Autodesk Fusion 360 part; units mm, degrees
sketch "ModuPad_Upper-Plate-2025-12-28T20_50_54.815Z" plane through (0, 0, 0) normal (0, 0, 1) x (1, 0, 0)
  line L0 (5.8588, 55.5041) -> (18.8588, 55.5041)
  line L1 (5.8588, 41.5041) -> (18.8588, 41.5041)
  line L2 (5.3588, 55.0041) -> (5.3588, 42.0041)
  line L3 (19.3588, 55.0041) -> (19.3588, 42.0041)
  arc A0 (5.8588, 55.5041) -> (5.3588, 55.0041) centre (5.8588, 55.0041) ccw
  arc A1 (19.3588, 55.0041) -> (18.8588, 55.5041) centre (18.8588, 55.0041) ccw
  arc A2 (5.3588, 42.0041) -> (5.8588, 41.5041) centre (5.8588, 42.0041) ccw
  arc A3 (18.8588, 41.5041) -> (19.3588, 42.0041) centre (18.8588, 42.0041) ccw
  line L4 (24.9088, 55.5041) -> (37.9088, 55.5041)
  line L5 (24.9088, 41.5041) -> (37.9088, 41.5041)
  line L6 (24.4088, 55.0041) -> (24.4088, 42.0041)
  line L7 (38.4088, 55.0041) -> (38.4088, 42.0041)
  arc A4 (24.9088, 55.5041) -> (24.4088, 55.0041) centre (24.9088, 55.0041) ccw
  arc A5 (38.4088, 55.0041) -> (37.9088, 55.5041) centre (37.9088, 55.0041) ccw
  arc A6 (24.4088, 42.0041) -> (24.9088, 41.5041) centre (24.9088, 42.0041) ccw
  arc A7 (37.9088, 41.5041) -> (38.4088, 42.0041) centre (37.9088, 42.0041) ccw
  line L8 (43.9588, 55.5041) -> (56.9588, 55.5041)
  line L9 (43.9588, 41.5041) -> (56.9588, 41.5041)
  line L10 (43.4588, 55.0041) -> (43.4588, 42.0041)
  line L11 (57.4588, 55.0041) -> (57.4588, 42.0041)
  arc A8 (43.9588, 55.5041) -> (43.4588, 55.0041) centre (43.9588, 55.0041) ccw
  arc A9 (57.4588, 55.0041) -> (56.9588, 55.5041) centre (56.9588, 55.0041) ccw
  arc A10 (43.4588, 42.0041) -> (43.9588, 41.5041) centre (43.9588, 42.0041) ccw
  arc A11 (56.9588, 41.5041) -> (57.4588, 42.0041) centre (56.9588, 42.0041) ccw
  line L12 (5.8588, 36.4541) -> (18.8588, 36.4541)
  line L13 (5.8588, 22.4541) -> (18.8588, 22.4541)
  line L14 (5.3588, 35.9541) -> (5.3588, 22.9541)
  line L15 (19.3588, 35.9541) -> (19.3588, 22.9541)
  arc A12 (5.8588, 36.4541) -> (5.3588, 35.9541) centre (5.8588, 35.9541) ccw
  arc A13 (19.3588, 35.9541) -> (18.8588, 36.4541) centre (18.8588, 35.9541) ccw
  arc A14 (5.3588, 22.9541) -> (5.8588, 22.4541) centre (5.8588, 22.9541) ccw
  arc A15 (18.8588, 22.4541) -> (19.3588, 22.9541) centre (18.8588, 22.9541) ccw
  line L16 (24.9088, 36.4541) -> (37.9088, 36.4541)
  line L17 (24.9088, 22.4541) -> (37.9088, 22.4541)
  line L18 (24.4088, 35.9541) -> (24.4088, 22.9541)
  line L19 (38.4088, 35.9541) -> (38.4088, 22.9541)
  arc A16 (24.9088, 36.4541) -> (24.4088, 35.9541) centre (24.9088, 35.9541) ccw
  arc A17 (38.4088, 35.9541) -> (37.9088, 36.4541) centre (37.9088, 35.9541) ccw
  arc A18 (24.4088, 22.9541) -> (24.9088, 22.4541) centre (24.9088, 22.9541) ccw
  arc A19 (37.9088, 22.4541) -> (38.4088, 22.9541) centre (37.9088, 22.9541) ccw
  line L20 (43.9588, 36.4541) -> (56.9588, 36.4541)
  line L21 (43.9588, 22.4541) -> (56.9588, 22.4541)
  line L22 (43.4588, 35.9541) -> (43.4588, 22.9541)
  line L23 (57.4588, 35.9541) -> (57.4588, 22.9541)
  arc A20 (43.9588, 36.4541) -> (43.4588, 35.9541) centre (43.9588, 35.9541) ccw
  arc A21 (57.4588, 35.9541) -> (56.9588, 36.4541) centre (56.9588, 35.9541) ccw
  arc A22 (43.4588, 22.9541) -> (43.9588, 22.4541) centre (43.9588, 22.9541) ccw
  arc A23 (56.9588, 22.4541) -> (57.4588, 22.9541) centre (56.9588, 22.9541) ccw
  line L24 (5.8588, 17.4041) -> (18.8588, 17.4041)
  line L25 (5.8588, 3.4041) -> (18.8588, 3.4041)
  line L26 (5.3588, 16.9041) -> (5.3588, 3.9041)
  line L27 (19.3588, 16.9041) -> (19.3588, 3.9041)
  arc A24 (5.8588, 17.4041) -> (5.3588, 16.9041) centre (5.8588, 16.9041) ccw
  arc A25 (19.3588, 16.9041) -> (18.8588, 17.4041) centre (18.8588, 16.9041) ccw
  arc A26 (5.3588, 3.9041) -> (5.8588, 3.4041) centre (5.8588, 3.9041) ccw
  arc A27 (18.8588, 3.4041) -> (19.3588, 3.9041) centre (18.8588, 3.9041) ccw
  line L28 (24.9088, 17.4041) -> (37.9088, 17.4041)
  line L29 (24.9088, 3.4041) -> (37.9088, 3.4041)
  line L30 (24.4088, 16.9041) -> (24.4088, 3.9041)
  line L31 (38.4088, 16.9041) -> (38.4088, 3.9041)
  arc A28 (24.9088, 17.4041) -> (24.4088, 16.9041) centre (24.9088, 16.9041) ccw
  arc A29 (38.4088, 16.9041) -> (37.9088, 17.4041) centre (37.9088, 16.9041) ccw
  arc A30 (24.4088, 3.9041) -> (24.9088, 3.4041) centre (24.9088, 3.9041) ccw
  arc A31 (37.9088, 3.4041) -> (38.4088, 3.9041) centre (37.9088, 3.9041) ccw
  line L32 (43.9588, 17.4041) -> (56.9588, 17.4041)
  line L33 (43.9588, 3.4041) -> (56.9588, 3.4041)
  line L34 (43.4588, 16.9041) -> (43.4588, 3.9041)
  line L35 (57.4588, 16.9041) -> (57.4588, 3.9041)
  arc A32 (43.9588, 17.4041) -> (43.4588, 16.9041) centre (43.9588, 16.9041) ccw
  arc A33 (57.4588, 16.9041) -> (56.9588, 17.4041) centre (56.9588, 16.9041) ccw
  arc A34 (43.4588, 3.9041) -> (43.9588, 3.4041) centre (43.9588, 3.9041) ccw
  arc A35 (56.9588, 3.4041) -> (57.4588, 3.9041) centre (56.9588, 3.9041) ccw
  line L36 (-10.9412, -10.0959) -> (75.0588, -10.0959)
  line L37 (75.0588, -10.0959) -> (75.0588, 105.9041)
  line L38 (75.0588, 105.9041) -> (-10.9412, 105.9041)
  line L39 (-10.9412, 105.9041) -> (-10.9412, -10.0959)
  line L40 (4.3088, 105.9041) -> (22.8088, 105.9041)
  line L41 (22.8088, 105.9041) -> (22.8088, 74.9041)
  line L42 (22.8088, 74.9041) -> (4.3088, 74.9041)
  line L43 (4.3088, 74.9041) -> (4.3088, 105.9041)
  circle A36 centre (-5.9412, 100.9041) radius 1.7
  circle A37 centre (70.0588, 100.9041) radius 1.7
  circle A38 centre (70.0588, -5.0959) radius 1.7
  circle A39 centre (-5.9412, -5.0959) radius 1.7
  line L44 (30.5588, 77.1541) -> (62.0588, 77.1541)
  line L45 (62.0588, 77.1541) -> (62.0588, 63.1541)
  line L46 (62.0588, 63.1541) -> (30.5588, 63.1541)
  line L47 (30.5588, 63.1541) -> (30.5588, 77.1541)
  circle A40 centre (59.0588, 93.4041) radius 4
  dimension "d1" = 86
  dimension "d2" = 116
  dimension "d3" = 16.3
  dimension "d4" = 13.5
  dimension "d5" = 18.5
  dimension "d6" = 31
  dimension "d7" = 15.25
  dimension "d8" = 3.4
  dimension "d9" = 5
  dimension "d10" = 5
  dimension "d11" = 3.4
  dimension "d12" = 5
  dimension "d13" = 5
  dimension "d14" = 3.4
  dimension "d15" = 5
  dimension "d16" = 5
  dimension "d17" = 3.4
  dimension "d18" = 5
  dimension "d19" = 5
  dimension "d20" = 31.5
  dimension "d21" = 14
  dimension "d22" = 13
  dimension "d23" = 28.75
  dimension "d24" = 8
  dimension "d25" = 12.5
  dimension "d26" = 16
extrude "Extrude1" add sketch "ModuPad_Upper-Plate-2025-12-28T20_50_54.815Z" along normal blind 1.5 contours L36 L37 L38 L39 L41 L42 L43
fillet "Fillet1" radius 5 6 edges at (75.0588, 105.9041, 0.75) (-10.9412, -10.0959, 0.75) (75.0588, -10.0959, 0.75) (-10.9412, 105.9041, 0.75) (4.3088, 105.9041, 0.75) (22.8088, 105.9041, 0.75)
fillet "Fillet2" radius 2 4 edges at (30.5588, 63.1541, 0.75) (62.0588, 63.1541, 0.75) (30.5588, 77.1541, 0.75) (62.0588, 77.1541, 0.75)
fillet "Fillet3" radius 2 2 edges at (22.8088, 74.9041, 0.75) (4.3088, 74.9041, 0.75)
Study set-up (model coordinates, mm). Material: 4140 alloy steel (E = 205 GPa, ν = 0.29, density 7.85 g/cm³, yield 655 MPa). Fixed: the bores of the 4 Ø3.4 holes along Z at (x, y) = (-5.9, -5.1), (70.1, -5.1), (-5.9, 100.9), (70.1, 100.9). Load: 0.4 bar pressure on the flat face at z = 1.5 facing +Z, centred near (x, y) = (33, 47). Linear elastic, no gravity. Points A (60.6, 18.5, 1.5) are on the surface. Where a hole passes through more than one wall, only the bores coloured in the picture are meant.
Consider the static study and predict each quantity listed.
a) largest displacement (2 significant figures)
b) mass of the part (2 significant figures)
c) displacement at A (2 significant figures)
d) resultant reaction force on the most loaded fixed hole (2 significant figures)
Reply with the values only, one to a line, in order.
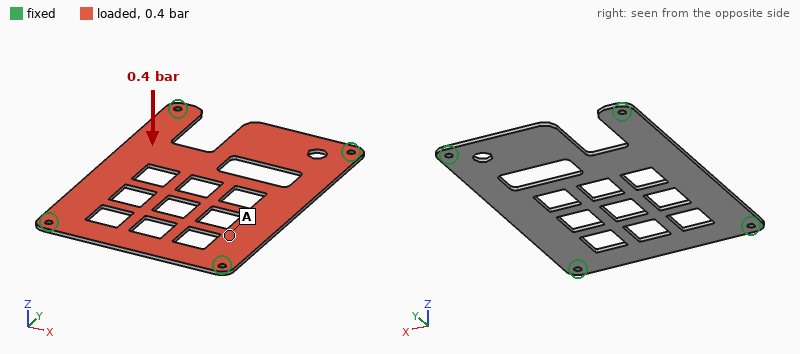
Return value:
0.44 mm
83 g
0.18 mm
80 N
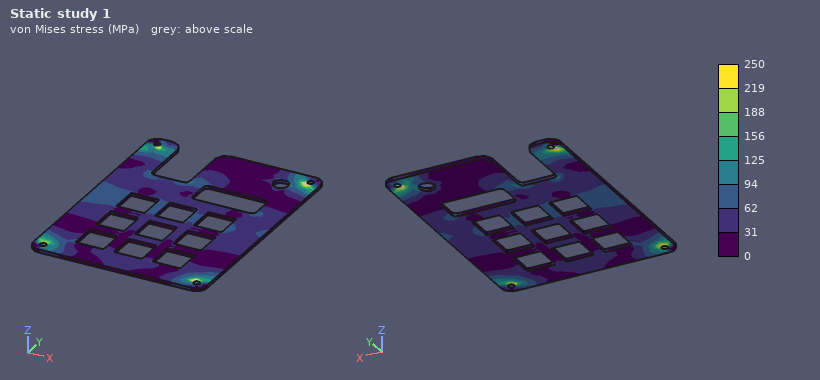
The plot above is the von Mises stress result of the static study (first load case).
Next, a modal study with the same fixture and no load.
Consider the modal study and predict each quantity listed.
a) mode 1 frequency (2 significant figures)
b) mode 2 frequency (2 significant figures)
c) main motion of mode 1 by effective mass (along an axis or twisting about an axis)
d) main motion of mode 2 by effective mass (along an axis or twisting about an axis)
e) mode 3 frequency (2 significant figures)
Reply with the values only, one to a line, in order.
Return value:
540 Hz
810 Hz
along Z
twisting about Y
960 Hz
